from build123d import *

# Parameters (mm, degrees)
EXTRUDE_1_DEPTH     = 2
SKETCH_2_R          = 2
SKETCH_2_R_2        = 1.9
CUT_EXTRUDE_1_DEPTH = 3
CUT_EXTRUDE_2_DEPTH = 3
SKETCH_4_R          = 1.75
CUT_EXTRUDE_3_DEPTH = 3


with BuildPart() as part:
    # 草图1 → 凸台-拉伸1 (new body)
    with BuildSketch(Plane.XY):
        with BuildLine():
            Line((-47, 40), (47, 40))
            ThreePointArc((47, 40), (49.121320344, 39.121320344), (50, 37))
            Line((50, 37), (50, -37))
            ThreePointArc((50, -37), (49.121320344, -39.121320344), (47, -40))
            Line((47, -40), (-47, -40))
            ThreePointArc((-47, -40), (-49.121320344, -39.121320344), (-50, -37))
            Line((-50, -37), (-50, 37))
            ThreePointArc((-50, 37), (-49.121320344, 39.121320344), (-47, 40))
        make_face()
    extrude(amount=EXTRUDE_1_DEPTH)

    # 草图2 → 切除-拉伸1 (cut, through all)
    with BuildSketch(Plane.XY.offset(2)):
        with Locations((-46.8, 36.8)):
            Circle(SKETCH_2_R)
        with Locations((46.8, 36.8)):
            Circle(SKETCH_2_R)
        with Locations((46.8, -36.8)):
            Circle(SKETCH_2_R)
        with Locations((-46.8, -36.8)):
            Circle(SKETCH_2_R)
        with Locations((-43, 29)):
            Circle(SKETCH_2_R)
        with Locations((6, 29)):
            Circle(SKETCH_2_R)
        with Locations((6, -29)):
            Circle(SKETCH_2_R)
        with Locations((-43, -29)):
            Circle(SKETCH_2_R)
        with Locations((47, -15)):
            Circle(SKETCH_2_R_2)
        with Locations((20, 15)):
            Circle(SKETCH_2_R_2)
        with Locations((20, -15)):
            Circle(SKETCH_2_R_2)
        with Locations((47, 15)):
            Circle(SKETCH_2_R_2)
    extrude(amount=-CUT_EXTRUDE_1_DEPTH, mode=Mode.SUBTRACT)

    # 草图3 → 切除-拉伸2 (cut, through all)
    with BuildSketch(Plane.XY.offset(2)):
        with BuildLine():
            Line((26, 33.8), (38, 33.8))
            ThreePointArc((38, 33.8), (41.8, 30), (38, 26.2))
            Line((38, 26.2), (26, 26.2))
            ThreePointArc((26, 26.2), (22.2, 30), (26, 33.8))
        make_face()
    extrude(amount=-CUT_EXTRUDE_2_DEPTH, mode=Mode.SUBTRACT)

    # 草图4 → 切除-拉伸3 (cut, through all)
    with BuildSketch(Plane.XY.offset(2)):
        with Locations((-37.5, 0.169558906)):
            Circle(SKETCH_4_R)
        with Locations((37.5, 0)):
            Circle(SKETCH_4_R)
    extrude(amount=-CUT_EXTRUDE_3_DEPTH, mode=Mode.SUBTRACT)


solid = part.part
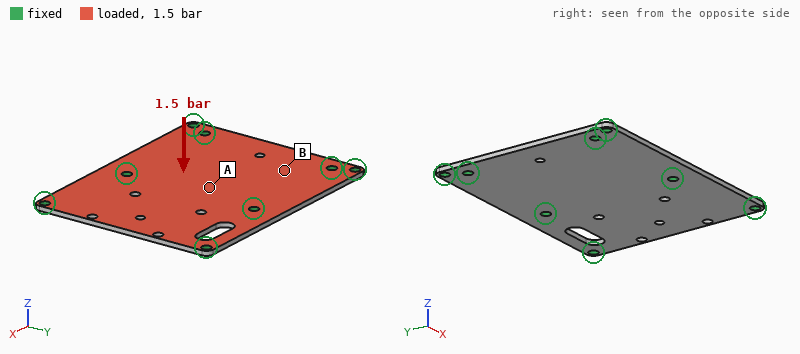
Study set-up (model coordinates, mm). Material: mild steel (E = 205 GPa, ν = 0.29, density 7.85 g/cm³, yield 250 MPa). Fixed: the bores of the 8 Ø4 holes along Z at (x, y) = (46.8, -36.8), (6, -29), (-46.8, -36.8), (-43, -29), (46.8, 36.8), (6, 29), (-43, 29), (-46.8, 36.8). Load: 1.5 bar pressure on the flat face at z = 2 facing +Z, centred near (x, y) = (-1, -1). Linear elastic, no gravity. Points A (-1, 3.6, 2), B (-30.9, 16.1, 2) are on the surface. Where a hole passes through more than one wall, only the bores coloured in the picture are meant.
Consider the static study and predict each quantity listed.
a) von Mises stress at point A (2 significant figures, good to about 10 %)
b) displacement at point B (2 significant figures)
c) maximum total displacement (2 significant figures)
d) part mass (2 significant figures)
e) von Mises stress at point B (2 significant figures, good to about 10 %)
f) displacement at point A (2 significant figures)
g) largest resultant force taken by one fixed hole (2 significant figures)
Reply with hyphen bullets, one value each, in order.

- 38 MPa
- 31 µm
- 91 µm
- 120 g
- 14 MPa
- 48 µm
- 290 N
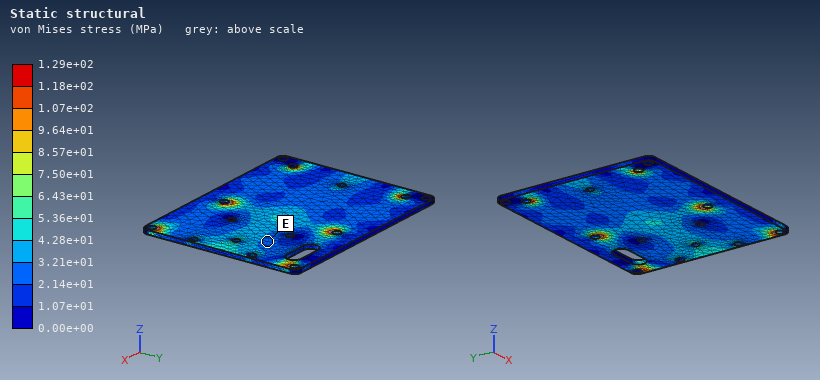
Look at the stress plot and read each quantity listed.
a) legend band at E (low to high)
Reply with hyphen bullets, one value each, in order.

- 2.14e+01 to 3.21e+01 MPa
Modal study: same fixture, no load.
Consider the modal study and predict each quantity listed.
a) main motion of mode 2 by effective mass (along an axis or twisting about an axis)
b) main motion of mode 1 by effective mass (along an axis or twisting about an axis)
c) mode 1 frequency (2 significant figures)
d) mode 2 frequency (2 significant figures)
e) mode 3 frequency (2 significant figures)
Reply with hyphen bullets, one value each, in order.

- along Z
- along Z
- 2100 Hz
- 2600 Hz
- 3900 Hz
